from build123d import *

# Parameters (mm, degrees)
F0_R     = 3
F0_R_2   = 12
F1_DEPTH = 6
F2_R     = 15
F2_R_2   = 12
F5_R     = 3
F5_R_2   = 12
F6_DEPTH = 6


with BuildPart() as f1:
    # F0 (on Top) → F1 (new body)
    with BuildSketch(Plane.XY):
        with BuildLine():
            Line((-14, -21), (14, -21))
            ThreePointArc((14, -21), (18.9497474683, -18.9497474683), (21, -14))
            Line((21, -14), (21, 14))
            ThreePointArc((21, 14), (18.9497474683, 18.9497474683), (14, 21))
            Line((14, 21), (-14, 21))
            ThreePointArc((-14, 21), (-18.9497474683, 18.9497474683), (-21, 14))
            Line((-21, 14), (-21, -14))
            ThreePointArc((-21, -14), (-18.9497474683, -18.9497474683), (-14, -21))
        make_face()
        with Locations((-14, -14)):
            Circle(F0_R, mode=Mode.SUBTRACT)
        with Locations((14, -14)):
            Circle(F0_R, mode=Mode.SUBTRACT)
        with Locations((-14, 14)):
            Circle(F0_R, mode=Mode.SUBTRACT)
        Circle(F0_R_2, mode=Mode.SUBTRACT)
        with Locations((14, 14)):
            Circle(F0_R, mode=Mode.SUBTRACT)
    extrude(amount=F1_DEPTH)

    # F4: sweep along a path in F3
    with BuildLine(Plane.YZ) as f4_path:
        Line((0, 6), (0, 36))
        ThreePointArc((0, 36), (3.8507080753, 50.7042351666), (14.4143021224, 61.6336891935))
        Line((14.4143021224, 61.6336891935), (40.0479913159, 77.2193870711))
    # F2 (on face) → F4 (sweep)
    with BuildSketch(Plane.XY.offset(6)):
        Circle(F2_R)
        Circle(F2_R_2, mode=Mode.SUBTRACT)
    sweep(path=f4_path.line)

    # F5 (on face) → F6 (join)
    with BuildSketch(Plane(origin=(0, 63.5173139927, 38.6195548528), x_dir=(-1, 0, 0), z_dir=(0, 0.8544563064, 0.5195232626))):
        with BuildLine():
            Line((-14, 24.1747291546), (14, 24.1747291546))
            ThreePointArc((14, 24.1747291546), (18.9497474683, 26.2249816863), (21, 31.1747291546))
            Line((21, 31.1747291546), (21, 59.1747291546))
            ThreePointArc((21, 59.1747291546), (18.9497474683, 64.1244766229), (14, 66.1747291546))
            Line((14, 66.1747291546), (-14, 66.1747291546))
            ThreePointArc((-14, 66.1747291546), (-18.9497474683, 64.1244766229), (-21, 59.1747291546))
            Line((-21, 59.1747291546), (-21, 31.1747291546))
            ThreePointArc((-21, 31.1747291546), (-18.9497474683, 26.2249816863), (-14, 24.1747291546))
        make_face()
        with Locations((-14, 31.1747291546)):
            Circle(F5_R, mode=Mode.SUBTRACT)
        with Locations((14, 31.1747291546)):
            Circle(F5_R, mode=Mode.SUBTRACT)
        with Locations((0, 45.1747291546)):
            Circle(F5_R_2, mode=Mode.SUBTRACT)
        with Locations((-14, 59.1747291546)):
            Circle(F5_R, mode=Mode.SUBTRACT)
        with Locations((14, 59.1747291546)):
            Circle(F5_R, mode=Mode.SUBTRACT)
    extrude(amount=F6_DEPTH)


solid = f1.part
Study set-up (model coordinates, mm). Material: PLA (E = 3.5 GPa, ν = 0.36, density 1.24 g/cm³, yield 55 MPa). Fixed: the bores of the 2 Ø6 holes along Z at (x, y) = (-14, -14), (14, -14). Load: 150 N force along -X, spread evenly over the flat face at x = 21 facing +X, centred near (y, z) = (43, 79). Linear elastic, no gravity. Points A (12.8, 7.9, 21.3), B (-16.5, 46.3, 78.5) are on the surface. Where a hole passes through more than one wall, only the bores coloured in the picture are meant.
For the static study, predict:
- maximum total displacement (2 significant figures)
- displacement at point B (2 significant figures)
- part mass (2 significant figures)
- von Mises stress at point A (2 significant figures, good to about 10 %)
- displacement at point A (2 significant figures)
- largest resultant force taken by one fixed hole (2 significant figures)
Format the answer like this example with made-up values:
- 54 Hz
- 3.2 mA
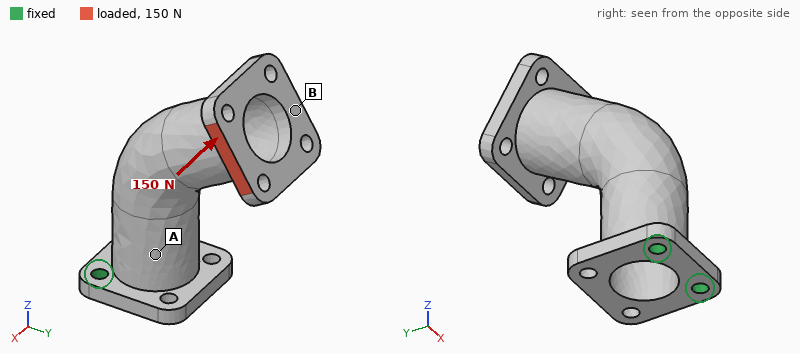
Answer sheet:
- 1.3 mm
- 1.1 mm
- 46 g
- 5.2 MPa
- 0.21 mm
- 520 N
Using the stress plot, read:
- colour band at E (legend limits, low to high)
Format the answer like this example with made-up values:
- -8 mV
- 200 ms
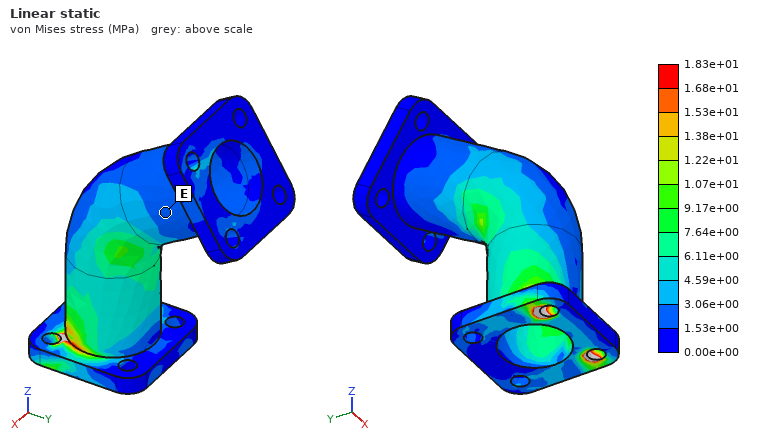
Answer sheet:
- 1.53e+00 to 3.06e+00 MPa
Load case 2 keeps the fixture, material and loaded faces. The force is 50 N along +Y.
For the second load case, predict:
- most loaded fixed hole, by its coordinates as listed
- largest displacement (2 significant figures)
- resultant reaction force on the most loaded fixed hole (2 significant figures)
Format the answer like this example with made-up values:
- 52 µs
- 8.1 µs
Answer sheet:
- (14, -14)
- 1.4 mm
- 59 N
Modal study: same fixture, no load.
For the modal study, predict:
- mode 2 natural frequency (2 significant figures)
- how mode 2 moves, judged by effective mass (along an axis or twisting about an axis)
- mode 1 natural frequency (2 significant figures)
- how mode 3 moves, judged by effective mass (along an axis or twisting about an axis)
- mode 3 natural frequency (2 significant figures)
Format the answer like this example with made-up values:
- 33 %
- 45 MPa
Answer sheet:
- 450 Hz
- along X
- 210 Hz
- twisting about Z
- 1400 Hz
